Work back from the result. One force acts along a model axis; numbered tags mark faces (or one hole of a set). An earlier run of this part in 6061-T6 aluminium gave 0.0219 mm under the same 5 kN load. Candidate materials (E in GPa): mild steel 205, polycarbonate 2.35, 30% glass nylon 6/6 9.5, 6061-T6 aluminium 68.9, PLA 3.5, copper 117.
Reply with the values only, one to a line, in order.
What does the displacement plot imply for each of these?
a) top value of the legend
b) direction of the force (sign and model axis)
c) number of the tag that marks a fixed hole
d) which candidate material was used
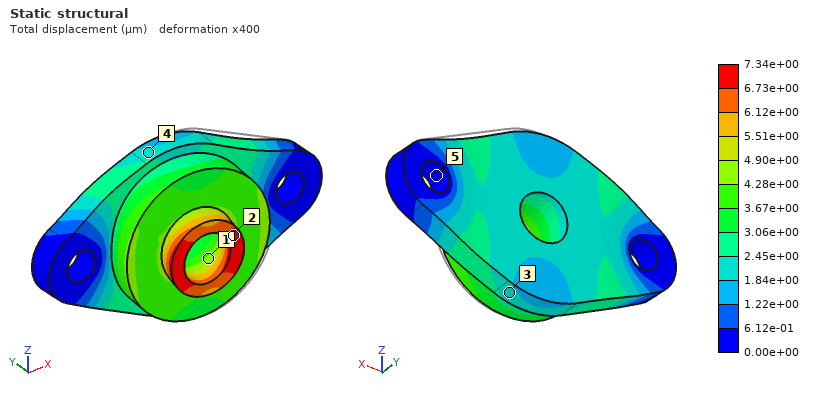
7.34e+00 µm
-X
5
mild steel
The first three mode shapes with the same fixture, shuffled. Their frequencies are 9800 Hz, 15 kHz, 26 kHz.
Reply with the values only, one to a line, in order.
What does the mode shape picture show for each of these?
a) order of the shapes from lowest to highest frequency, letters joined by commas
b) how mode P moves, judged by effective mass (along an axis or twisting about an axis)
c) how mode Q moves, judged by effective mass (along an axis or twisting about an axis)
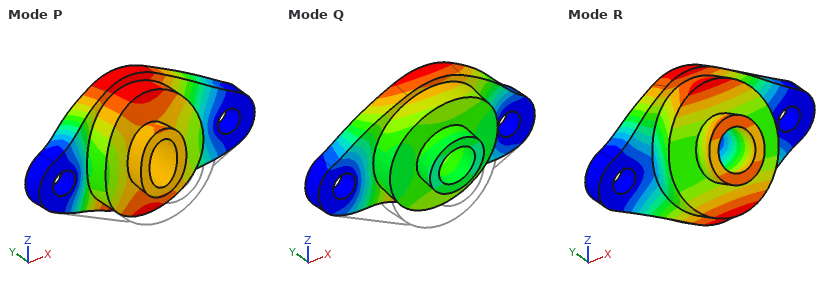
R, P, Q
along Y
along Z
